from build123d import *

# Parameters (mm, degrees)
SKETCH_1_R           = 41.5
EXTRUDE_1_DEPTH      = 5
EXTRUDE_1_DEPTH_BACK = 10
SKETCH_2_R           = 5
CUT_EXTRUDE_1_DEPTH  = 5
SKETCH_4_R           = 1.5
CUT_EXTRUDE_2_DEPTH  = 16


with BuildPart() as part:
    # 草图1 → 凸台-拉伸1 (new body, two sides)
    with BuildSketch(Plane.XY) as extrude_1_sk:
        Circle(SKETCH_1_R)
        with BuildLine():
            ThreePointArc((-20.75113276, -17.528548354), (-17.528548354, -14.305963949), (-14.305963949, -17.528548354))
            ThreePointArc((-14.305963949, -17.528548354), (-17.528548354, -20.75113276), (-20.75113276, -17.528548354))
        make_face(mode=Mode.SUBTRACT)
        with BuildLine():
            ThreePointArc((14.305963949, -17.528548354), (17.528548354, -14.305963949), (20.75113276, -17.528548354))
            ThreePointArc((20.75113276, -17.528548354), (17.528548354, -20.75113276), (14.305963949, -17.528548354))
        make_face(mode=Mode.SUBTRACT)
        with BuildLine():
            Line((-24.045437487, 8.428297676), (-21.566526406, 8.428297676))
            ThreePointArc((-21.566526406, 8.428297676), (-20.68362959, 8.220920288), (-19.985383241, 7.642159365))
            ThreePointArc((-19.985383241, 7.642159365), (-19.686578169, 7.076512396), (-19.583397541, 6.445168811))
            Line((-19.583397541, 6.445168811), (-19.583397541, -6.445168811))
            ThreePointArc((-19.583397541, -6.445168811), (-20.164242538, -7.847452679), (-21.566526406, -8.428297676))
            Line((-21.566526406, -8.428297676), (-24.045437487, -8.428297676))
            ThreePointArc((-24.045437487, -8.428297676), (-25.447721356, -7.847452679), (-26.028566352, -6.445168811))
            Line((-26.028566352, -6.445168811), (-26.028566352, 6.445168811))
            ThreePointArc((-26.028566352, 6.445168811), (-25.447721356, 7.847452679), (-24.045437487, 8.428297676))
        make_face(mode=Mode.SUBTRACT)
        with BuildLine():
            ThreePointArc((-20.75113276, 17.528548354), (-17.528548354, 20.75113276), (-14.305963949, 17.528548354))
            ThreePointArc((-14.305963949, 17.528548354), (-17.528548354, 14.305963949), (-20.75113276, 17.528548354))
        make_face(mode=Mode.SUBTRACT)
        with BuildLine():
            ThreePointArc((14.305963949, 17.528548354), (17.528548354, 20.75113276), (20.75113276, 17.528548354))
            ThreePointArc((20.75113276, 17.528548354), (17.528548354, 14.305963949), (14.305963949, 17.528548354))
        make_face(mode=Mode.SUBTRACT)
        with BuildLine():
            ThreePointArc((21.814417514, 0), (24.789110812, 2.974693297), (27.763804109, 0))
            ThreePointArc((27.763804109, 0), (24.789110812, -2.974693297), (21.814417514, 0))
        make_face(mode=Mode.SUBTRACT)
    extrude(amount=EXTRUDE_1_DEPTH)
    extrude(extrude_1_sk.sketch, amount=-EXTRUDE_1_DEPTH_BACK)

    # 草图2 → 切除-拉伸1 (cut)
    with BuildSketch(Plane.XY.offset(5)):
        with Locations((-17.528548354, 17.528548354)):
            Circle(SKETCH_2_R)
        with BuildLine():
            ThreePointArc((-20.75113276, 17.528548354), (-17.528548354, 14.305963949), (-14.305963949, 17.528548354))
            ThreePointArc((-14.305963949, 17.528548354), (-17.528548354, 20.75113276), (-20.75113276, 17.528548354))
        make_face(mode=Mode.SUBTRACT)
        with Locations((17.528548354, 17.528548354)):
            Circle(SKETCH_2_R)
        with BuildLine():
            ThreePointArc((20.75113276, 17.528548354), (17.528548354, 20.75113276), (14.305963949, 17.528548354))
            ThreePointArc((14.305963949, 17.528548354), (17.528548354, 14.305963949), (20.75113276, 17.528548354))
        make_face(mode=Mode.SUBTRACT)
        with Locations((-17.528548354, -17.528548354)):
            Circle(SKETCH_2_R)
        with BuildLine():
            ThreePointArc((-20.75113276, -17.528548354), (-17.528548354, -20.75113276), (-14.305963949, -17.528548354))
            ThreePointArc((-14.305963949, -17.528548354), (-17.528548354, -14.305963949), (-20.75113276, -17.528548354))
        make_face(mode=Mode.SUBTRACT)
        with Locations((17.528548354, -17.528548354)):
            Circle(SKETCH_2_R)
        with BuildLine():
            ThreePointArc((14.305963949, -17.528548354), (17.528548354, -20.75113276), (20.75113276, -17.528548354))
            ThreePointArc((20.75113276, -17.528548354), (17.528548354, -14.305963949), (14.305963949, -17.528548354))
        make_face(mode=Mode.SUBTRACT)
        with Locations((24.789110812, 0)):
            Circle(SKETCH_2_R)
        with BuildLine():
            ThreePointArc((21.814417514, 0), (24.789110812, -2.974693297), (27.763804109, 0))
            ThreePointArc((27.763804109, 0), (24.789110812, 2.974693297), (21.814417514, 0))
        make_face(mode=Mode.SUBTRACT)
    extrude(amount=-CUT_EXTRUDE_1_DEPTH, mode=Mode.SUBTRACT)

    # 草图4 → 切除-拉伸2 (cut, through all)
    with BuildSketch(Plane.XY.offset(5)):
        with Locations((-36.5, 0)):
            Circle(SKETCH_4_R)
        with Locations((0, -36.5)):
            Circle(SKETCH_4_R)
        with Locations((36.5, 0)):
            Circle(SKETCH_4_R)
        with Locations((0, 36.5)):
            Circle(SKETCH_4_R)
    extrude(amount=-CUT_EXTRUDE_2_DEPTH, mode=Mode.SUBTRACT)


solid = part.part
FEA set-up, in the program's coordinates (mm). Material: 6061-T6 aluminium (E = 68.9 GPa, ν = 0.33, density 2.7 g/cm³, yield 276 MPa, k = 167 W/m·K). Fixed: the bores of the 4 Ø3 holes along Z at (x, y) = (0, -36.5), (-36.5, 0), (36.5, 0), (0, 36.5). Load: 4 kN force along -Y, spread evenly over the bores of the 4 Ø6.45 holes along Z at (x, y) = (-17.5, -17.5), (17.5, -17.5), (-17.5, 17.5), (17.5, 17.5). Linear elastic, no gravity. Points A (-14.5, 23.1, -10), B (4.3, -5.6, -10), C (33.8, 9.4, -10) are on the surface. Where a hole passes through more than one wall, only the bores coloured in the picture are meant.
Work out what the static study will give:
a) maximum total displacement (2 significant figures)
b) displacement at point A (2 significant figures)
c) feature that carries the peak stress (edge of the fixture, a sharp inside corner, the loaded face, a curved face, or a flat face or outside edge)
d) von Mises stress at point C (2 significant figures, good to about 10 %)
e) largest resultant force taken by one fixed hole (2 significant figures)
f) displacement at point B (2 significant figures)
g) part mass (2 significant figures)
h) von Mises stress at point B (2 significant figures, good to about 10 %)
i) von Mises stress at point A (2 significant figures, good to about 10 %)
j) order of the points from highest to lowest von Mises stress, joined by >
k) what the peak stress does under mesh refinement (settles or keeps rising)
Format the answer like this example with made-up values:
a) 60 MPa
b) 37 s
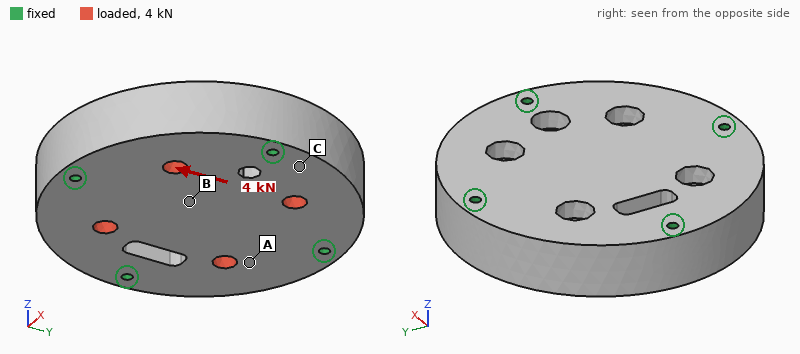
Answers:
a) 2.1 µm
b) 1.6 µm
c) edge of the fixture
d) 2.9 MPa
e) 1.1 kN
f) 1.4 µm
g) 200 g
h) 1.3 MPa
i) 4.8 MPa
j) A > C > B
k) keeps rising
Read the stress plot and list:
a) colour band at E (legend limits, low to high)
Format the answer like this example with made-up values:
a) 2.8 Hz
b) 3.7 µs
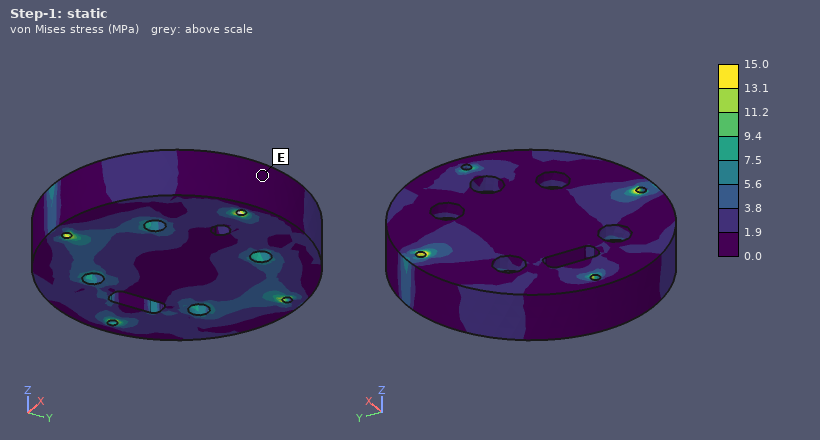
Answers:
a) 0.0 to 1.9 MPa
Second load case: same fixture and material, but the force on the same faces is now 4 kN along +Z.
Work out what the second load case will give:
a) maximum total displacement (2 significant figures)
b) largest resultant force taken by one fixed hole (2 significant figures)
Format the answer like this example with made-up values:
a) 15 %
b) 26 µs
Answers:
a) 6.1 µm
b) 1.0 kN
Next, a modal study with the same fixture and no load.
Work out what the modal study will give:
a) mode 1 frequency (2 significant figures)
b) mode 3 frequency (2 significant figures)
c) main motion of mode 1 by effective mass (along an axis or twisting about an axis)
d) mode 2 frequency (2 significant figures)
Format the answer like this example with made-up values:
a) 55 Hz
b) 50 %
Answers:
a) 12 kHz
b) 15 kHz
c) along Z
d) 15 kHz
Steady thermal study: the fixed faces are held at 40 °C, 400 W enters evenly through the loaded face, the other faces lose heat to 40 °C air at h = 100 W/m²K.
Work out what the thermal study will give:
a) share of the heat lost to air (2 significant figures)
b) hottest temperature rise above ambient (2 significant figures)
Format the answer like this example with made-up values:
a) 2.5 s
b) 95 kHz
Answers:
a) 7.7 %
b) 37 K
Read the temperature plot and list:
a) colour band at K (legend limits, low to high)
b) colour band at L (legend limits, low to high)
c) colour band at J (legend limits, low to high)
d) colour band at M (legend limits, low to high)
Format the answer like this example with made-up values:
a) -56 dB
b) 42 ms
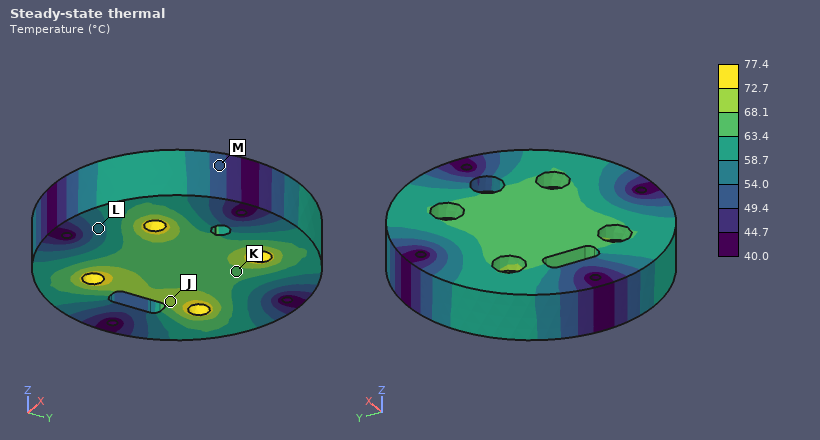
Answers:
a) 63.4 to 68.1 °C
b) 54.0 to 58.7 °C
c) 68.1 to 72.7 °C
d) 49.4 to 54.0 °C
